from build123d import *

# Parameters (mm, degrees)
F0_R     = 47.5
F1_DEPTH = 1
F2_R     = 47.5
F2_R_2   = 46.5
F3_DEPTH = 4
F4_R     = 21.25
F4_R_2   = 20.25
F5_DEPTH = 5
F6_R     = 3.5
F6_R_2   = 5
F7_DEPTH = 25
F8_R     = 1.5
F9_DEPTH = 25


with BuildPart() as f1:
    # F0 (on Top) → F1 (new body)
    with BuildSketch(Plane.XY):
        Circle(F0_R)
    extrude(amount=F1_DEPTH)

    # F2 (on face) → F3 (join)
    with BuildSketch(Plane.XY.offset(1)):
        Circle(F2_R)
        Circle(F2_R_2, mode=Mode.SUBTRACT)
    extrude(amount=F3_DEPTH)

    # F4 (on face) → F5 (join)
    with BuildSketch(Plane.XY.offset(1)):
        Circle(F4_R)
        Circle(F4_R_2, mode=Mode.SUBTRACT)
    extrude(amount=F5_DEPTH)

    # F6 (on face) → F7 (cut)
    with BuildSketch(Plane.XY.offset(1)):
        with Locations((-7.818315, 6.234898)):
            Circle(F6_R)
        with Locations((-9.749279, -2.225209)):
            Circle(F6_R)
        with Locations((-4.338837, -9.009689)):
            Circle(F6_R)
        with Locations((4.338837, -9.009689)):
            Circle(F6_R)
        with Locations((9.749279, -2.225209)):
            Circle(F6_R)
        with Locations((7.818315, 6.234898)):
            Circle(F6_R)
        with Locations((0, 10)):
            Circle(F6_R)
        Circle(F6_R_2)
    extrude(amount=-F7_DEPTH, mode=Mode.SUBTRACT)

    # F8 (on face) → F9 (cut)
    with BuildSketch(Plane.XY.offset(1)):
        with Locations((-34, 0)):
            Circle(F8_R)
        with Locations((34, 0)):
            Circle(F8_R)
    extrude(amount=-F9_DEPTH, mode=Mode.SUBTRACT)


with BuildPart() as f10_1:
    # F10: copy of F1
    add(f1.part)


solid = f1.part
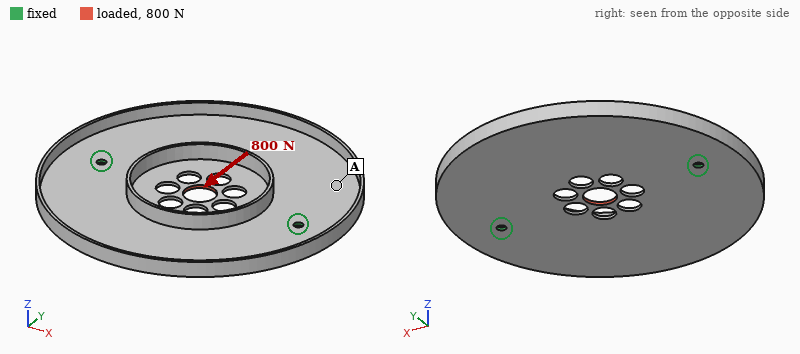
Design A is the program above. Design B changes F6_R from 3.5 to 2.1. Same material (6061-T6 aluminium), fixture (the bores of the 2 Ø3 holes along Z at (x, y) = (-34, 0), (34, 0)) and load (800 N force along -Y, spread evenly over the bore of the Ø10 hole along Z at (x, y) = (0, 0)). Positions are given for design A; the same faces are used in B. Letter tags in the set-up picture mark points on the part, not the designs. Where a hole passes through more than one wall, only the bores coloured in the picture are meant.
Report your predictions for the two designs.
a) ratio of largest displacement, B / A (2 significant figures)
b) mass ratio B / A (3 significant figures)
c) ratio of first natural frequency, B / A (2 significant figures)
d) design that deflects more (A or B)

0.67
1.02
1.00
A
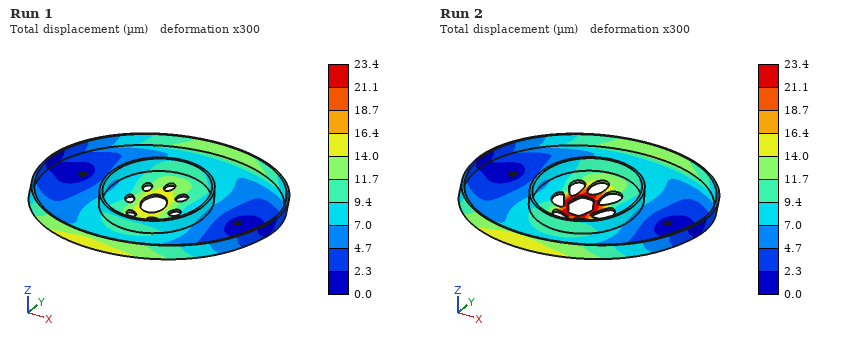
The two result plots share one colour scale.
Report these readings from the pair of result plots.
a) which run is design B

Run 1
